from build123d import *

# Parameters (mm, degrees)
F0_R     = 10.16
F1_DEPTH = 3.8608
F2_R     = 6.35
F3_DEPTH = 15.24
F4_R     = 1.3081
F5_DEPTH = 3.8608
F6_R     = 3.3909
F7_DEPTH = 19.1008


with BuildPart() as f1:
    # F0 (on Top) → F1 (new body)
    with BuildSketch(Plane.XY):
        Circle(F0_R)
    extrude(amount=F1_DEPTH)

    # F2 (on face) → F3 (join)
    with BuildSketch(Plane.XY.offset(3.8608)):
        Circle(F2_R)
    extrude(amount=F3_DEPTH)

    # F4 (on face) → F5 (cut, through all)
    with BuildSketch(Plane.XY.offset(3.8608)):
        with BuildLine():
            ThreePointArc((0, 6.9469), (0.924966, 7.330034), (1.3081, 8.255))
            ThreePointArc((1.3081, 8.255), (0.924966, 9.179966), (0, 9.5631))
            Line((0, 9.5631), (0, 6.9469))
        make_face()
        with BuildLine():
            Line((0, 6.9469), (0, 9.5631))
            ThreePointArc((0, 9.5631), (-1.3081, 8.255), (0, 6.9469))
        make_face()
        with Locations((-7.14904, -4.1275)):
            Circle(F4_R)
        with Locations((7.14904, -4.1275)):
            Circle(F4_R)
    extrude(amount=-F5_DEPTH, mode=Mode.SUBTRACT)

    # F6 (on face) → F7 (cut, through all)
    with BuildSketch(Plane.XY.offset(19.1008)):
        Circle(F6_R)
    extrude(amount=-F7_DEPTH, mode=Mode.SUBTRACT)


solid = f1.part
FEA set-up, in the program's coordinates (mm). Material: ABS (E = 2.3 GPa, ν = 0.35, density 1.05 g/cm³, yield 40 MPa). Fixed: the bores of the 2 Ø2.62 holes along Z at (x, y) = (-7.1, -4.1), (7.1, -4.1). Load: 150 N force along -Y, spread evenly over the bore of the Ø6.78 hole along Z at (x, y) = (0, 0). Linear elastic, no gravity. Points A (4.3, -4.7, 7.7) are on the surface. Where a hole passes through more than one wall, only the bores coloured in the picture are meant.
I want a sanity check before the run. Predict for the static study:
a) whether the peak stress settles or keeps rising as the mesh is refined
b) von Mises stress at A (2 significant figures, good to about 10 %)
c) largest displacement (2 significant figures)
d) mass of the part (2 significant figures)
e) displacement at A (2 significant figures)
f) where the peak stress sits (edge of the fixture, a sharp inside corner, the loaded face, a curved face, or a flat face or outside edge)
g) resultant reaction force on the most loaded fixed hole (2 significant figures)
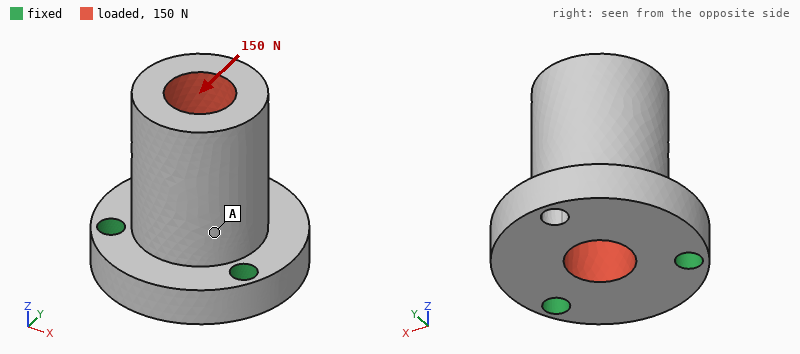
keeps rising
3.6 MPa
0.36 mm
2.6 g
0.10 mm
edge of the fixture
75 N
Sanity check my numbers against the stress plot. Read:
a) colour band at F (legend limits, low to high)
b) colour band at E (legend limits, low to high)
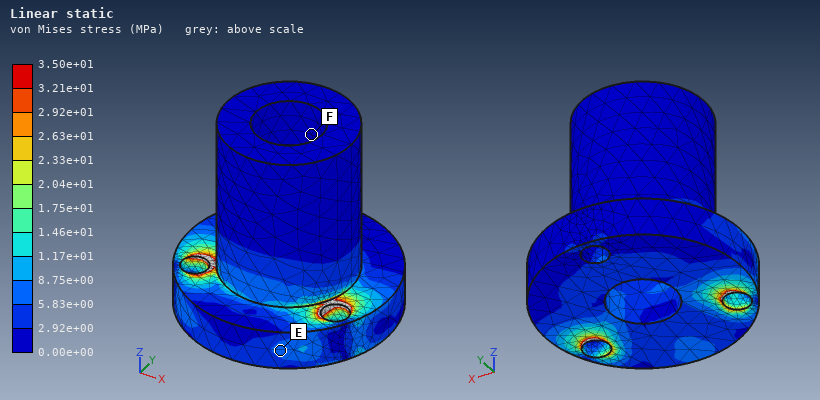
0.00e+00 to 2.92e+00 MPa
5.83e+00 to 8.75e+00 MPa
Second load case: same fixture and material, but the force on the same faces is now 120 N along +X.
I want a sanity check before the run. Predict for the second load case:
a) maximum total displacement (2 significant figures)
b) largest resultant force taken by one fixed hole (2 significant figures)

74 µm
96 N
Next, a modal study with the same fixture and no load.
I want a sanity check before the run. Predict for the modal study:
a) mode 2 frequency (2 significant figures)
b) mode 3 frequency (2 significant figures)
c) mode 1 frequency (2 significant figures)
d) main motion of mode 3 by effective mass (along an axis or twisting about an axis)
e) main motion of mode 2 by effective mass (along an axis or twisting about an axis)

5500 Hz
10 kHz
2600 Hz
along X
along X
